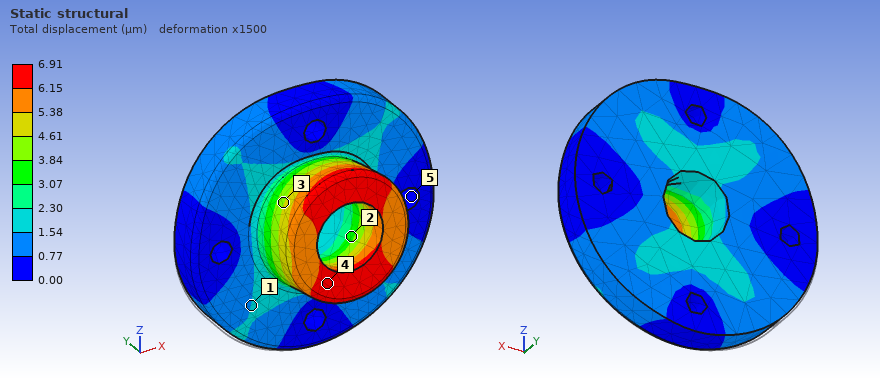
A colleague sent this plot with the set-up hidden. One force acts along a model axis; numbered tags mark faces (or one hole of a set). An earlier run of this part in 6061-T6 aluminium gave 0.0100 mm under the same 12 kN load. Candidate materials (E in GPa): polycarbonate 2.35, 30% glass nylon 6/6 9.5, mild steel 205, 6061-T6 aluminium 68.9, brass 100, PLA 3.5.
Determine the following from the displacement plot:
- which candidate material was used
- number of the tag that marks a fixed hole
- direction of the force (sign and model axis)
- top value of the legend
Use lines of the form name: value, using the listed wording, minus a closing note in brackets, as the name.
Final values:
which candidate material was used: brass
number of the tag that marks a fixed hole: 5
direction of the force: +Z
top value of the legend: 6.91 µm
